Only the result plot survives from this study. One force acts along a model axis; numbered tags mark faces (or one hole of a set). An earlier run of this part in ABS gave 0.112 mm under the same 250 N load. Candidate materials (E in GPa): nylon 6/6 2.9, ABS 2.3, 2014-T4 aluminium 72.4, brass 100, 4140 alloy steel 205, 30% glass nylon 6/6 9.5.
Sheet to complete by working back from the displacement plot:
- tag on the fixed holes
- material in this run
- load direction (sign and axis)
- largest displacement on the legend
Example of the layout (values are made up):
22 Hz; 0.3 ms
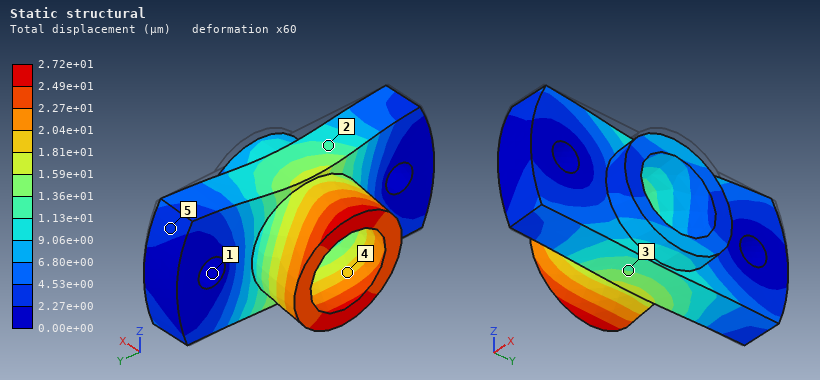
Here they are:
1; 30% glass nylon 6/6; -Z; 2.72e+01 µm
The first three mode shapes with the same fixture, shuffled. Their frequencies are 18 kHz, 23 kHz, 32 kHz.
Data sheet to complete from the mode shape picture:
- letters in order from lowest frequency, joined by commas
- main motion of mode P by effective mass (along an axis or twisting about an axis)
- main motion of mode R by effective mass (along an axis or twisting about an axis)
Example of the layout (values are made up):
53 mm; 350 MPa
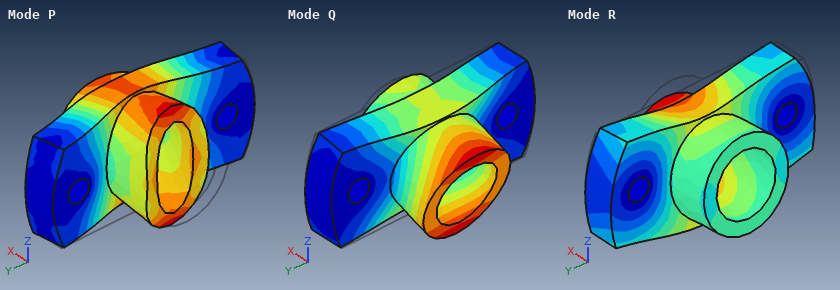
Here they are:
Q, P, R; along X; along Z
